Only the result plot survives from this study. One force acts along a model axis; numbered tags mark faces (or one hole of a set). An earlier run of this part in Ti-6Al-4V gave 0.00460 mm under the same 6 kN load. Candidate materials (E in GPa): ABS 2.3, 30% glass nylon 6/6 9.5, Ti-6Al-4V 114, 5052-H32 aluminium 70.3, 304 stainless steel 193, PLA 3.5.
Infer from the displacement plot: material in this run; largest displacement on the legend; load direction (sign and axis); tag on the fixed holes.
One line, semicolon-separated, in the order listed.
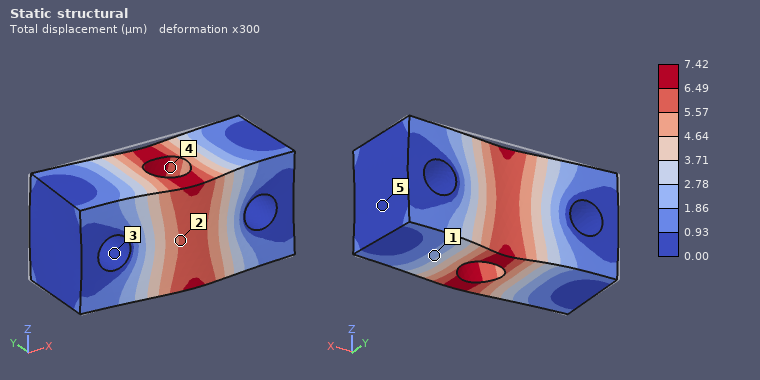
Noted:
5052-H32 aluminium; 7.42 µm; -Y; 3
